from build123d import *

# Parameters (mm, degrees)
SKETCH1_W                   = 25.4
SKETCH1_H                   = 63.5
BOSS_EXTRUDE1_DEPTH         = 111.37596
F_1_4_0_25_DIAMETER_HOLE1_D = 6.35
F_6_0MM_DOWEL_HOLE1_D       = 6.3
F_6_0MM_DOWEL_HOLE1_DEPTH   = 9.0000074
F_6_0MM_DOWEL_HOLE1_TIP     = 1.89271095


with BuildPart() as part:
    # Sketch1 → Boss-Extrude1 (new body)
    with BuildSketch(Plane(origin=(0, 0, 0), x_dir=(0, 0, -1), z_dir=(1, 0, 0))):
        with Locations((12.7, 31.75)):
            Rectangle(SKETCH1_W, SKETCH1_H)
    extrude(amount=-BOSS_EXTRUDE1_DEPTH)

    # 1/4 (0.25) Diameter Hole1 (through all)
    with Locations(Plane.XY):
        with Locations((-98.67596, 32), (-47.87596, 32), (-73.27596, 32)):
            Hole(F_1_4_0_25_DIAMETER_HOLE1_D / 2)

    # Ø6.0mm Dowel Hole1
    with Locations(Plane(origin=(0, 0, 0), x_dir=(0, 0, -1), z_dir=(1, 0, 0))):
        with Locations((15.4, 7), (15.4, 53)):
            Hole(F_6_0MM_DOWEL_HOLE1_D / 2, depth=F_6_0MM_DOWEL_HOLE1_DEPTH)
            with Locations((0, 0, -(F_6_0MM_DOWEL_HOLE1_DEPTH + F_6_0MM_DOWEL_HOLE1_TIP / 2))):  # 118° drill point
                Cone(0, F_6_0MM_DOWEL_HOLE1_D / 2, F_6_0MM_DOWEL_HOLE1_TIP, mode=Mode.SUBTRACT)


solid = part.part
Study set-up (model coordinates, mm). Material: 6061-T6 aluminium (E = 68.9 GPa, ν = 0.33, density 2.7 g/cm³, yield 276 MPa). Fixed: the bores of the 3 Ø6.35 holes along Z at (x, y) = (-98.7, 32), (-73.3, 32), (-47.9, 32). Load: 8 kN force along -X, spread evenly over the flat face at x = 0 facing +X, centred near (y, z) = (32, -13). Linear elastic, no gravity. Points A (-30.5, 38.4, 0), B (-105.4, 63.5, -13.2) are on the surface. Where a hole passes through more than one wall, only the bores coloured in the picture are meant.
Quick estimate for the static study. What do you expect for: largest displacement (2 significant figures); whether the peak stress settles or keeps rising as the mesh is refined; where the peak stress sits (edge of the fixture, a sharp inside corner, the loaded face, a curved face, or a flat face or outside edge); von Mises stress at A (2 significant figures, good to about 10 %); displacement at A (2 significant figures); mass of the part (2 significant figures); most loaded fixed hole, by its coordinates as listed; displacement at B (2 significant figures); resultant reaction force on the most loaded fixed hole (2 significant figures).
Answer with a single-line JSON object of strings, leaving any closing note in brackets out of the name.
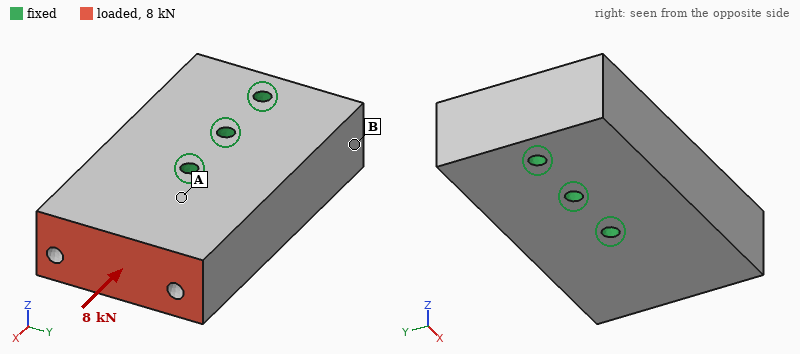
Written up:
{"largest displacement": "5.1 µm", "whether the peak stress settles or keeps rising as the mesh is refined": "keeps rising", "where the peak stress sits": "edge of the fixture", "von Mises stress at A": "6.8 MPa", "displacement at A": "2.3 µm", "mass of the part": "480 g", "most loaded fixed hole, by its coordinates as listed": "(-47.9, 32)", "displacement at B": "0.83 µm", "resultant reaction force on the most loaded fixed hole": "5.2 kN"}
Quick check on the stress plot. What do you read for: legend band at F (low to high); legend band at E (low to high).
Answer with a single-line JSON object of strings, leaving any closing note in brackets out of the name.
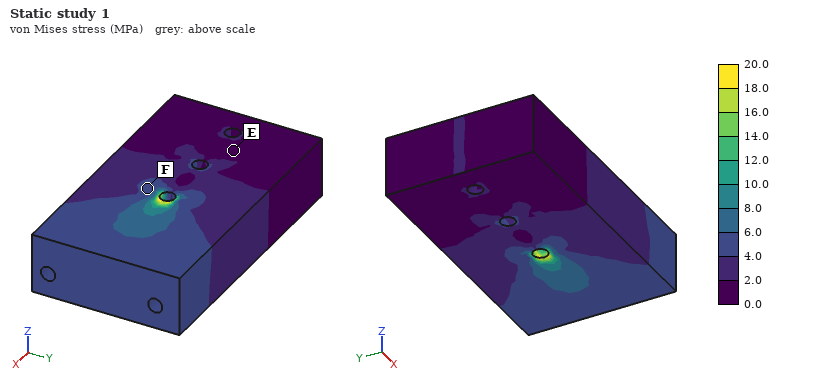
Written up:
{"legend band at F": "4.0 to 6.0 MPa", "legend band at E": "0.0 to 2.0 MPa"}
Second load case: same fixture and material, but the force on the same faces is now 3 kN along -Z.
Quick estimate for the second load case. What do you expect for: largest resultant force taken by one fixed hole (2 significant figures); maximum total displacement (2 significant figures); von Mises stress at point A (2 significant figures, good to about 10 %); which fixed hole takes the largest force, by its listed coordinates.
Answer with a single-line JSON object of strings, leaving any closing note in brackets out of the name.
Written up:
{"largest resultant force taken by one fixed hole": "4.5 kN", "maximum total displacement": "34 µm", "von Mises stress at point A": "14 MPa", "which fixed hole takes the largest force, by its listed coordinates": "(-47.9, 32)"}
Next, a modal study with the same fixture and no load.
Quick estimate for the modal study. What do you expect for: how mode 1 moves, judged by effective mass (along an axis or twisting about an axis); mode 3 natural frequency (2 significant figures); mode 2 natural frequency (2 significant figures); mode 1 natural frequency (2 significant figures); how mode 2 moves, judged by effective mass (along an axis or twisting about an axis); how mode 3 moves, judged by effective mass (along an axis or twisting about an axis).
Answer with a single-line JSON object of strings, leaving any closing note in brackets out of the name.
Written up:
{"how mode 1 moves, judged by effective mass": "along Z", "mode 3 natural frequency": "8300 Hz", "mode 2 natural frequency": "7600 Hz", "mode 1 natural frequency": "6000 Hz", "how mode 2 moves, judged by effective mass": "along Y", "how mode 3 moves, judged by effective mass": "twisting about X"}
